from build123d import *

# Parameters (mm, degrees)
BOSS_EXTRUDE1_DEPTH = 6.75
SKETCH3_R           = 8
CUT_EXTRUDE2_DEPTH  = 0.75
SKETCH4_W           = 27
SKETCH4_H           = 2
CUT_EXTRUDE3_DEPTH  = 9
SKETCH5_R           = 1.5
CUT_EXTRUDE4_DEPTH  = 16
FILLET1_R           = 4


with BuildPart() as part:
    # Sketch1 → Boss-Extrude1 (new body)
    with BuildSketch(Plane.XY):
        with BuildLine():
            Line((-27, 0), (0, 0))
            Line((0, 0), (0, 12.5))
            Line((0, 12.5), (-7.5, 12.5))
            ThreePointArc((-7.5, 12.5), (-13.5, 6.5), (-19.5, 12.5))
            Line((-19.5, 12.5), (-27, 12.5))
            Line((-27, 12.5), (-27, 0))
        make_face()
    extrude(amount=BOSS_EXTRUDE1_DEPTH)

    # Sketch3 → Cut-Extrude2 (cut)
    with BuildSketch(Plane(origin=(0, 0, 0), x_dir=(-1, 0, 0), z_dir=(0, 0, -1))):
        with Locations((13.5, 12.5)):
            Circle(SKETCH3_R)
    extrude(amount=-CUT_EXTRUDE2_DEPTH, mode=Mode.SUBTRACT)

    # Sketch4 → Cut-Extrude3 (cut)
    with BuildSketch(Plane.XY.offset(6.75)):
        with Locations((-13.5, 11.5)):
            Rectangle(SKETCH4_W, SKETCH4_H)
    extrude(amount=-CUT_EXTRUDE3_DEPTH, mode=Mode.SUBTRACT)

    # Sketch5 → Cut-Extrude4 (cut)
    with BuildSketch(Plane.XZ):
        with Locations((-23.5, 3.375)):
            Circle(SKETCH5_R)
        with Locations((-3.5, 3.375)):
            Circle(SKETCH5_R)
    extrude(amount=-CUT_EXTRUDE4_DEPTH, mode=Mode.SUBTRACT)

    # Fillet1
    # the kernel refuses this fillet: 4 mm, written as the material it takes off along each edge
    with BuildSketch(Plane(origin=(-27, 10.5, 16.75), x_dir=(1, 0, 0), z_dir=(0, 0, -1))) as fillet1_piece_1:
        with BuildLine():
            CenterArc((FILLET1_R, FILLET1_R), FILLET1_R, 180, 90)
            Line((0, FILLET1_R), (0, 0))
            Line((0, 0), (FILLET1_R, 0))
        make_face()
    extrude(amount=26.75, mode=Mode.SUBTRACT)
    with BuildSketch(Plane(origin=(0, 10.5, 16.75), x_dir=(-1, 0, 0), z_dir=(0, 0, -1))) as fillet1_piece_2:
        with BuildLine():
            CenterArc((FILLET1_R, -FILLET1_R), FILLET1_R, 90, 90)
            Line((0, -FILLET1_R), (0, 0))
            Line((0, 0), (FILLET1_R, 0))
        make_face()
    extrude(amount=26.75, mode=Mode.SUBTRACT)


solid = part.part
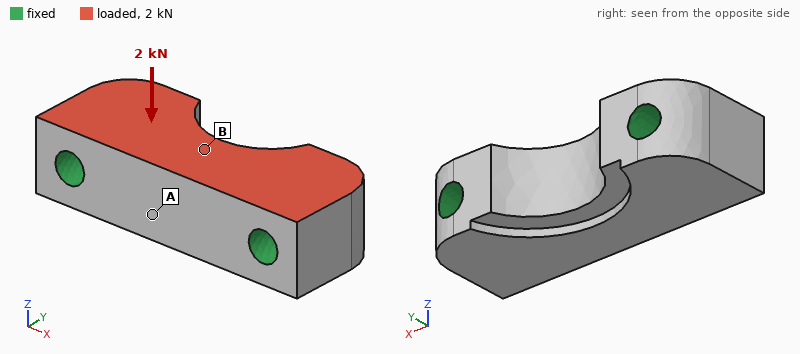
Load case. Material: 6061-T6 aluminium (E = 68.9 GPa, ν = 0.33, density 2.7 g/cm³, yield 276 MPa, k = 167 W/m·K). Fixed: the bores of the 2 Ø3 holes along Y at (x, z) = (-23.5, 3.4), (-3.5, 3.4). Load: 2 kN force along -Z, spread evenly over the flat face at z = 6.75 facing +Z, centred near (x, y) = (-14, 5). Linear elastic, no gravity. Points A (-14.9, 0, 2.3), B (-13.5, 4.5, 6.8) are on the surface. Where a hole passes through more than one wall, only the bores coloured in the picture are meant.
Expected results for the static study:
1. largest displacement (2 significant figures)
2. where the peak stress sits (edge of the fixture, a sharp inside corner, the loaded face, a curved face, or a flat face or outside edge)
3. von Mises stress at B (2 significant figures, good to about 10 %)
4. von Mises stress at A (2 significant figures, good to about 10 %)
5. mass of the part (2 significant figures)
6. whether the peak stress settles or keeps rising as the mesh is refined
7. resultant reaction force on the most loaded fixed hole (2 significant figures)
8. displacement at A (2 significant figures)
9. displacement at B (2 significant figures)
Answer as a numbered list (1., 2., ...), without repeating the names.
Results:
1. 5.0 µm
2. edge of the fixture
3. 21 MPa
4. 8.0 MPa
5. 4.0 g
6. keeps rising
7. 1.0 kN
8. 4.5 µm
9. 4.1 µm
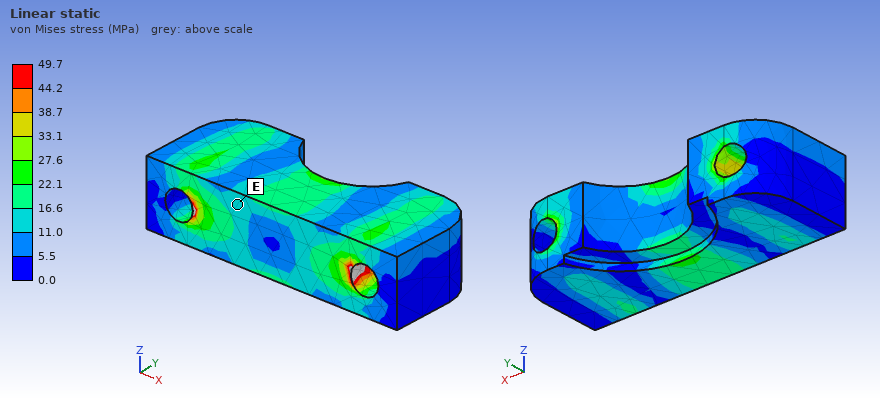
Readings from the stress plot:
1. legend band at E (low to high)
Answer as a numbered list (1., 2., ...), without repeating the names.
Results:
1. 11.0 to 16.6 MPa
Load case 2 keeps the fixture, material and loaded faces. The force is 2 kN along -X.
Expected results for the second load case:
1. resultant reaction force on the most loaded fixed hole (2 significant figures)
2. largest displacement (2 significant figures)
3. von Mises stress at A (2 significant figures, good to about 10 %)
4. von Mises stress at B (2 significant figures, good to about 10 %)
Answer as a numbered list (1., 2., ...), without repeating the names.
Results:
1. 1.0 kN
2. 2.0 µm
3. 3.9 MPa
4. 15 MPa
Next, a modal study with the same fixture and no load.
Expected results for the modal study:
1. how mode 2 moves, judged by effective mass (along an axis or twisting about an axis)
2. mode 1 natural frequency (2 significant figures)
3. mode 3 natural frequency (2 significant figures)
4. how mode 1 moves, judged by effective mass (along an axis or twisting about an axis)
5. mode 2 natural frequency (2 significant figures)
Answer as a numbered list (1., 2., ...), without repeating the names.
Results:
1. along Y
2. 59 kHz
3. 97 kHz
4. along Z
5. 78 kHz
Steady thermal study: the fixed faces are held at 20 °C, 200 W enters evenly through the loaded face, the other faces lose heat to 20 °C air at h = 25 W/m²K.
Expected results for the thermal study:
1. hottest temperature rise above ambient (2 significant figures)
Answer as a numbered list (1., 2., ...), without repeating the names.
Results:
1. 40 K
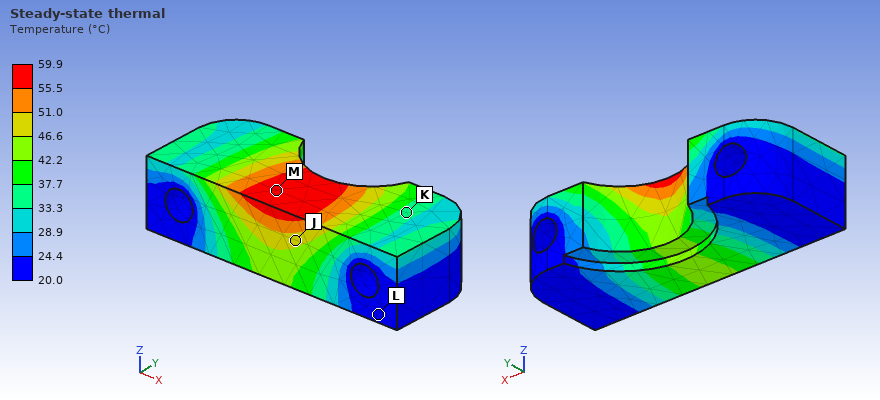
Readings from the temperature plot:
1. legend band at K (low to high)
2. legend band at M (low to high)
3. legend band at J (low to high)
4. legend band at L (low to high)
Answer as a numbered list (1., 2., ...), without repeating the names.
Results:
1. 33.3 to 37.7 °C
2. 55.5 to 59.9 °C
3. 46.6 to 51.0 °C
4. 20.0 to 24.4 °C
